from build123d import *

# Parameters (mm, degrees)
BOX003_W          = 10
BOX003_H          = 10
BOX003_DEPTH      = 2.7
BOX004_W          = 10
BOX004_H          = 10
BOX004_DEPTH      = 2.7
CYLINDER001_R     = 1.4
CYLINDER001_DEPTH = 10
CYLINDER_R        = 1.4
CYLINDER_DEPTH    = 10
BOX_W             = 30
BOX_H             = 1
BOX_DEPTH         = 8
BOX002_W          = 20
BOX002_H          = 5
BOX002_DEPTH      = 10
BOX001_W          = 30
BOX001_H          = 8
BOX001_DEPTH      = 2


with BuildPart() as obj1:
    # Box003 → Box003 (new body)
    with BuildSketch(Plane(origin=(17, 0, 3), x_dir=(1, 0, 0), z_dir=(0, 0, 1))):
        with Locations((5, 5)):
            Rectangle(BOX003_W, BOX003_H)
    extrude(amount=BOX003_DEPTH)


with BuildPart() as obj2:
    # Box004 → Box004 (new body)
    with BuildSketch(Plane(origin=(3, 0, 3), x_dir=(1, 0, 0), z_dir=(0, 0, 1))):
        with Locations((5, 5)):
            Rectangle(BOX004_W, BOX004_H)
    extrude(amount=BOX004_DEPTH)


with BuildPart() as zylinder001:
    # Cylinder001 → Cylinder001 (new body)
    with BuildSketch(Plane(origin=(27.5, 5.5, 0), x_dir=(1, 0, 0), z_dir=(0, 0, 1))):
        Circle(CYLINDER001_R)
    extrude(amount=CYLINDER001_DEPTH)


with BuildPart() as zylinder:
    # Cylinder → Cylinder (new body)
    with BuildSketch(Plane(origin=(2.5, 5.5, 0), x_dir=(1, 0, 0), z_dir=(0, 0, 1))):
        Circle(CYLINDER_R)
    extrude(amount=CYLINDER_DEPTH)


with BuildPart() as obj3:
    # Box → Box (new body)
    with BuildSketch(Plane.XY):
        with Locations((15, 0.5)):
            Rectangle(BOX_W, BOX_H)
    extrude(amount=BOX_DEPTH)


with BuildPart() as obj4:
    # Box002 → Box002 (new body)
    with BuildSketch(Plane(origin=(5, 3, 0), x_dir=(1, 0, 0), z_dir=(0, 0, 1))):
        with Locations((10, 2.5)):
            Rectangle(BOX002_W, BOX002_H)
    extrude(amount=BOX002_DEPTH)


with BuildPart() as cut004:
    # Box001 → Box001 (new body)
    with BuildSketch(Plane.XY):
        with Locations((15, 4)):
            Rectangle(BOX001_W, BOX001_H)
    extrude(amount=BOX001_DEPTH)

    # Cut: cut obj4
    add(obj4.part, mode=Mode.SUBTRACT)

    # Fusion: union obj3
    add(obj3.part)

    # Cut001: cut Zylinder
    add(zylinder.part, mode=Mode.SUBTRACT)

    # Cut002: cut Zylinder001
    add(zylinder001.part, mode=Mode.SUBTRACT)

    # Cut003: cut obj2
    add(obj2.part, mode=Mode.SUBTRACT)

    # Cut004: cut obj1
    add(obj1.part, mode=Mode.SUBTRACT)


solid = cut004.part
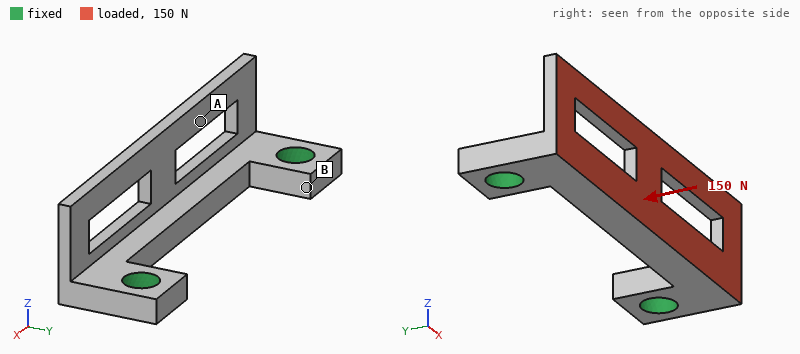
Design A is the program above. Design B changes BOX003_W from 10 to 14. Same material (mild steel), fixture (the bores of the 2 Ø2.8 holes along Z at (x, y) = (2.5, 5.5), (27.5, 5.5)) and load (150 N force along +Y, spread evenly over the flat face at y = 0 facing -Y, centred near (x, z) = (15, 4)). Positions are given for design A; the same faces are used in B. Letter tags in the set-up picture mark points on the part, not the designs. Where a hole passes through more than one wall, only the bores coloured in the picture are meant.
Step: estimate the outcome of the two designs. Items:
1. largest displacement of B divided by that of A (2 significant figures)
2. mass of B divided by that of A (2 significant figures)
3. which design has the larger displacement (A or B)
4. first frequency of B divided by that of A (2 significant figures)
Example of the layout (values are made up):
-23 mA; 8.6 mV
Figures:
1.7; 0.97; B; 0.80
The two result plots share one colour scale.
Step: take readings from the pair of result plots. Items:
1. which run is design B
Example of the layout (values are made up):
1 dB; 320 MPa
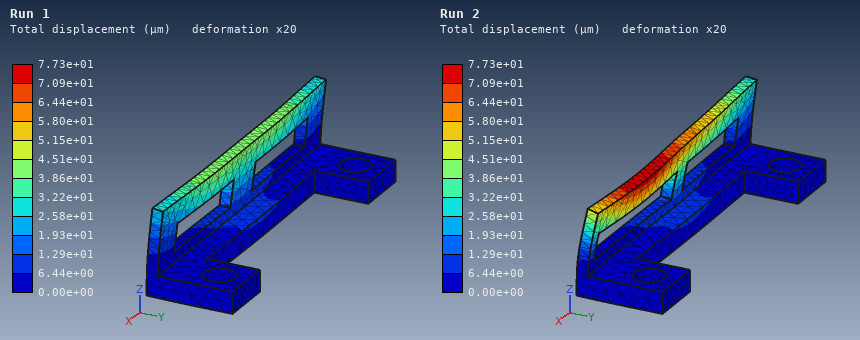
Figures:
Run 2
